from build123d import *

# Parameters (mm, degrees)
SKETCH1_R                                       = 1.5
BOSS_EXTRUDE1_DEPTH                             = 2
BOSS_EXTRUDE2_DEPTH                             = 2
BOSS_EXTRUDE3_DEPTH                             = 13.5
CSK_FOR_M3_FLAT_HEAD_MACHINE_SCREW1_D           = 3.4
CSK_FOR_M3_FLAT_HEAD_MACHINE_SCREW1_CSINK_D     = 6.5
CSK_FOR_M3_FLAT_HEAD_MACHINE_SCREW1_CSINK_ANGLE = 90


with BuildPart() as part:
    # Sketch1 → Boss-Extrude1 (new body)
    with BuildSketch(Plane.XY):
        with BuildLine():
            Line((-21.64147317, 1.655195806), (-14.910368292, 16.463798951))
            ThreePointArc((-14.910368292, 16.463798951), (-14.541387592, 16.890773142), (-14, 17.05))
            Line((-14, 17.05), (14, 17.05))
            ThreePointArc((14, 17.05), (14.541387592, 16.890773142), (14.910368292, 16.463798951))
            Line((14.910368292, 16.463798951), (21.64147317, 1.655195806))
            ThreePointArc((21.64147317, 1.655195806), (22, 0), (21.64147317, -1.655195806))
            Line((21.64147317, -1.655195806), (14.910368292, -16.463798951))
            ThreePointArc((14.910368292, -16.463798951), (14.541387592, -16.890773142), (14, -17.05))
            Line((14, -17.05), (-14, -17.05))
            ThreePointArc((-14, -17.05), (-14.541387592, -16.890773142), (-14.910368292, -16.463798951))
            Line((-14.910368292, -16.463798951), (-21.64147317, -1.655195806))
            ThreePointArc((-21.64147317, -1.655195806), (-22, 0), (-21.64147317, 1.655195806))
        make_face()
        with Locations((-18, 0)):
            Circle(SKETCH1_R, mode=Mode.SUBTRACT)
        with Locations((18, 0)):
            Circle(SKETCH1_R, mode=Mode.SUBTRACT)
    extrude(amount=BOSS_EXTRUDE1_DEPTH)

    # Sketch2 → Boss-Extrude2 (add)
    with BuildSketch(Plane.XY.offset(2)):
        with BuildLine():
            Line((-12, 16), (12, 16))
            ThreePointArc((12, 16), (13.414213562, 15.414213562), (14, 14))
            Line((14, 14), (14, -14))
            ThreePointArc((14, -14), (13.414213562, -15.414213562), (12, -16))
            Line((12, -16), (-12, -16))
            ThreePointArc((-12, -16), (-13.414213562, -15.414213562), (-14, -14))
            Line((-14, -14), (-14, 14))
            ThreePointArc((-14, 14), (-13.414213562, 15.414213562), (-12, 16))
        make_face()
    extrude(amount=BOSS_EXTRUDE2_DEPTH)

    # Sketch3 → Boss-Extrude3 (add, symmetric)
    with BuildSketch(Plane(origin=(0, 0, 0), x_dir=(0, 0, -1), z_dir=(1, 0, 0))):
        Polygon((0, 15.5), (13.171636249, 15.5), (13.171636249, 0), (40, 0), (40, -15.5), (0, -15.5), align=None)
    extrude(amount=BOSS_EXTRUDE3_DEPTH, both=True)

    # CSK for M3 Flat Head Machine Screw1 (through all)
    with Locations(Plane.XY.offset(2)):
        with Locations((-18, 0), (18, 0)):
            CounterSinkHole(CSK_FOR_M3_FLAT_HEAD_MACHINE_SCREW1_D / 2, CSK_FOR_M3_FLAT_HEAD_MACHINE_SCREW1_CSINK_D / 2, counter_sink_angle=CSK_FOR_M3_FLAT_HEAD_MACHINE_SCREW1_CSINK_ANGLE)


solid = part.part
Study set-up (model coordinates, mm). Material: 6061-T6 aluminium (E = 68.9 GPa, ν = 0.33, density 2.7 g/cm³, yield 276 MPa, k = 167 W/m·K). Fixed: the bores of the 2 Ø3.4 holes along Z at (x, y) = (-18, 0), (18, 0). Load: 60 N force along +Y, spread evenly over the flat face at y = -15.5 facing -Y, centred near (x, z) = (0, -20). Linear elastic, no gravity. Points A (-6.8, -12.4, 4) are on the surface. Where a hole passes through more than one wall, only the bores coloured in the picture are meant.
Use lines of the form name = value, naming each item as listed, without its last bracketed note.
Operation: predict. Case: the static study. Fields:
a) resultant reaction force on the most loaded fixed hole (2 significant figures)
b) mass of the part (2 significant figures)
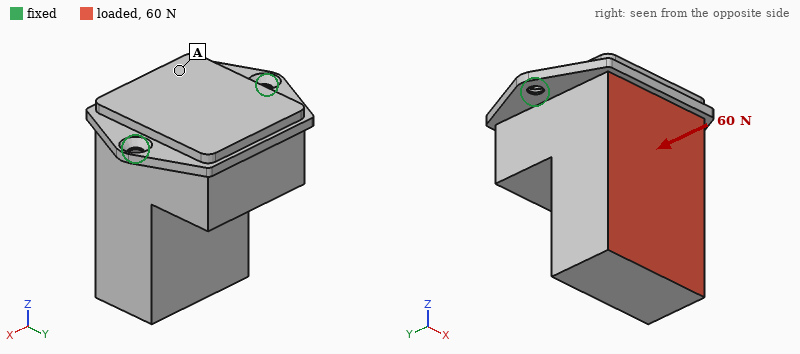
resultant reaction force on the most loaded fixed hole = 30 N
mass of the part = 72 g
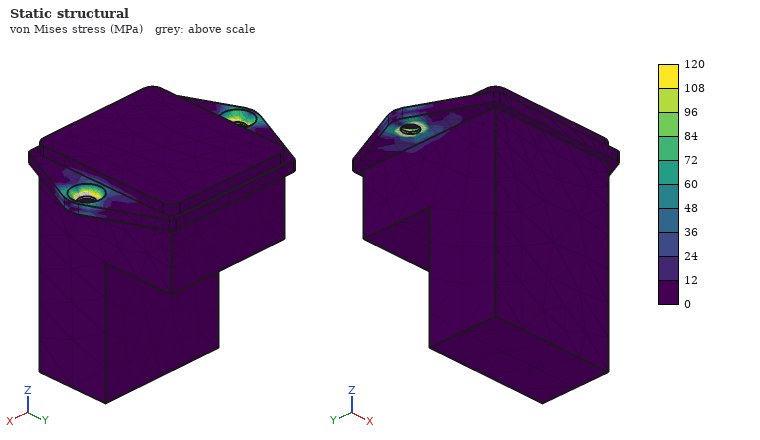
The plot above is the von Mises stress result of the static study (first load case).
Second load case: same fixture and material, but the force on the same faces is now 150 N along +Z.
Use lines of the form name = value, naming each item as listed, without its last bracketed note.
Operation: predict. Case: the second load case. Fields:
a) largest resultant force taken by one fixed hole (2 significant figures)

largest resultant force taken by one fixed hole = 90 N
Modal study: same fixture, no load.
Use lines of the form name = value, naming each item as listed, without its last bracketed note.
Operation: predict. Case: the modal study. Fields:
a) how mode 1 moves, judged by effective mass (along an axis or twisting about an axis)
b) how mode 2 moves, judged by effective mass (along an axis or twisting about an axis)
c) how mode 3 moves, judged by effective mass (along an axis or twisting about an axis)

how mode 1 moves, judged by effective mass = along Y
how mode 2 moves, judged by effective mass = along X
how mode 3 moves, judged by effective mass = along Z
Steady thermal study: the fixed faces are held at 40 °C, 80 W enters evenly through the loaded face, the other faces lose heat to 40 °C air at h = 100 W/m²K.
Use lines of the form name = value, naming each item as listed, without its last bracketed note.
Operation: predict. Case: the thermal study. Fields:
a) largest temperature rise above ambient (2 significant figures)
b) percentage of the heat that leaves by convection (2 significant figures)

largest temperature rise above ambient = 64 K
percentage of the heat that leaves by convection = 35 %
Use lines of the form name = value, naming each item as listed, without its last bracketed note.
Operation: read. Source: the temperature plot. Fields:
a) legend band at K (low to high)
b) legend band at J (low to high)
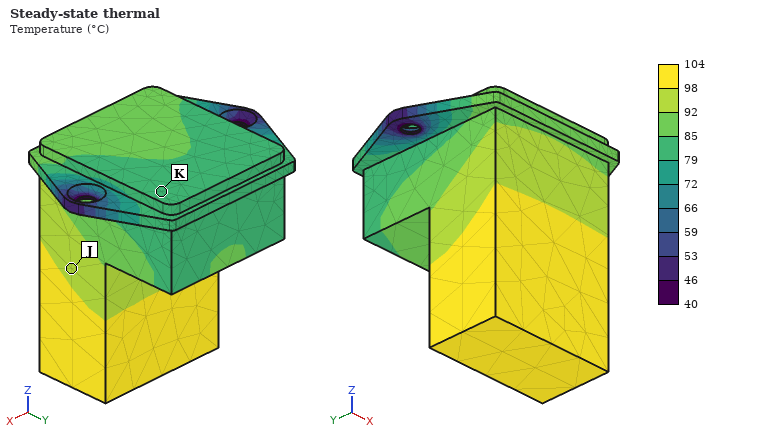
legend band at K = 79 to 85 °C
legend band at J = 92 to 98 °C
